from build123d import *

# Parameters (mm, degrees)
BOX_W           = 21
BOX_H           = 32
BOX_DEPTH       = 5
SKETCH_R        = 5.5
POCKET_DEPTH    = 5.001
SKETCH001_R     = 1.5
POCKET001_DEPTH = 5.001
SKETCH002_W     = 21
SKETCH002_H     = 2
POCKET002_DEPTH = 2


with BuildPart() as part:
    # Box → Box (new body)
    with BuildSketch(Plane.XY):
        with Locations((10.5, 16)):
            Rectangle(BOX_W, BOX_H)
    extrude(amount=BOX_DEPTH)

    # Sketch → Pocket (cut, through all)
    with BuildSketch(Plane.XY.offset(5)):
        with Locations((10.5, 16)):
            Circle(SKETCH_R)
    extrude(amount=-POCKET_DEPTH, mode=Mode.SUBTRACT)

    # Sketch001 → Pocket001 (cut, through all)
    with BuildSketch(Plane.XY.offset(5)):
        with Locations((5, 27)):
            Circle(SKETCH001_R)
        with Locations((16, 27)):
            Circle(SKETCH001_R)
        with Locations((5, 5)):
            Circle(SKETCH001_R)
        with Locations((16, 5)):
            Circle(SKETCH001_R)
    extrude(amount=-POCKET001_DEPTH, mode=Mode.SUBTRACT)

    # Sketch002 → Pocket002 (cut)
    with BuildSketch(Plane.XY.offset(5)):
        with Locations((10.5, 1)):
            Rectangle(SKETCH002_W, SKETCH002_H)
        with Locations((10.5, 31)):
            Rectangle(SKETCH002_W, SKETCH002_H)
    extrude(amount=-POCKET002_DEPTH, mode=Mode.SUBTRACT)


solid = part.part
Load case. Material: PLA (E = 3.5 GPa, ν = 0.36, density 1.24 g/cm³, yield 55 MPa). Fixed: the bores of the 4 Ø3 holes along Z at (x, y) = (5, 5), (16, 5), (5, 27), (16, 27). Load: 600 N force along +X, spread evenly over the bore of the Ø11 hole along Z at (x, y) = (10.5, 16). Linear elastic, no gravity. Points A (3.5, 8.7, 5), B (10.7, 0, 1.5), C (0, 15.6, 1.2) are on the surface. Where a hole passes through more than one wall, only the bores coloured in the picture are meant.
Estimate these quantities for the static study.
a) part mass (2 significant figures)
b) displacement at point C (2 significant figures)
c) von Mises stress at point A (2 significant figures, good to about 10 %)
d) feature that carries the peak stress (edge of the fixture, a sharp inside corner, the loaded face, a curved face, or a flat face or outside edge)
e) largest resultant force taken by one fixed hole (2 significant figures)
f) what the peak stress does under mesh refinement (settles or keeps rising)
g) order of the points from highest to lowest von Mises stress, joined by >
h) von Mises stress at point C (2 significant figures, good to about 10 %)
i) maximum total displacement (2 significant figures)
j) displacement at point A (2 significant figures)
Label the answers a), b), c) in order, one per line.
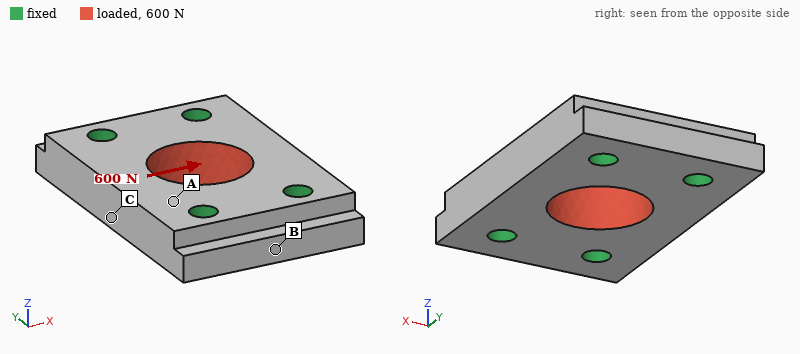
a) 3.2 g
b) 26 µm
c) 4.2 MPa
d) edge of the fixture
e) 160 N
f) keeps rising
g) C > A > B
h) 8.3 MPa
i) 31 µm
j) 9.3 µm
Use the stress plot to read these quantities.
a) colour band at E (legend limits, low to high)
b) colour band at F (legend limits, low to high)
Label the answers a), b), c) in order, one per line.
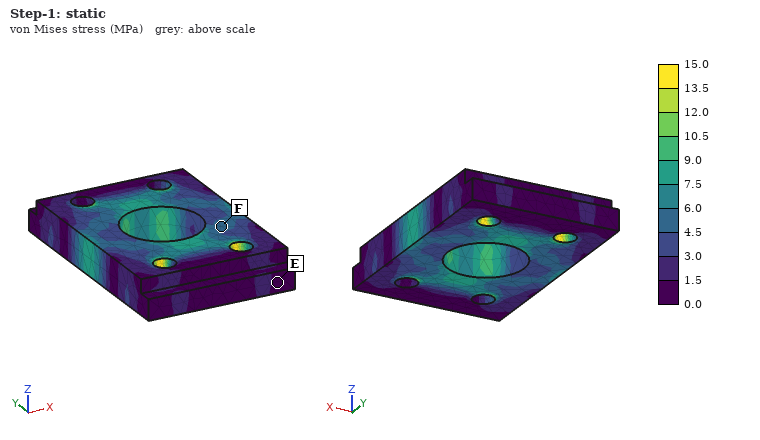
a) 0.0 to 1.5 MPa
b) 4.5 to 6.0 MPa
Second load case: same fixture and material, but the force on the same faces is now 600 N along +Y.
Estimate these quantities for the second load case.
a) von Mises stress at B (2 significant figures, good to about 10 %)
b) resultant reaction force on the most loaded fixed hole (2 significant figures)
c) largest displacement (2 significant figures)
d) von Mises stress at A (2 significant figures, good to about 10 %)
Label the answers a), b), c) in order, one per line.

a) 1.3 MPa
b) 150 N
c) 10 µm
d) 2.8 MPa
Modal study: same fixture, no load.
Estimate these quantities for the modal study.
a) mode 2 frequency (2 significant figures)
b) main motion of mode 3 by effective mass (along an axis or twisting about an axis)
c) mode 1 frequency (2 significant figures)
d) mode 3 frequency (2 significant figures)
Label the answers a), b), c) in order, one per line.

a) 16 kHz
b) along X
c) 15 kHz
d) 23 kHz
